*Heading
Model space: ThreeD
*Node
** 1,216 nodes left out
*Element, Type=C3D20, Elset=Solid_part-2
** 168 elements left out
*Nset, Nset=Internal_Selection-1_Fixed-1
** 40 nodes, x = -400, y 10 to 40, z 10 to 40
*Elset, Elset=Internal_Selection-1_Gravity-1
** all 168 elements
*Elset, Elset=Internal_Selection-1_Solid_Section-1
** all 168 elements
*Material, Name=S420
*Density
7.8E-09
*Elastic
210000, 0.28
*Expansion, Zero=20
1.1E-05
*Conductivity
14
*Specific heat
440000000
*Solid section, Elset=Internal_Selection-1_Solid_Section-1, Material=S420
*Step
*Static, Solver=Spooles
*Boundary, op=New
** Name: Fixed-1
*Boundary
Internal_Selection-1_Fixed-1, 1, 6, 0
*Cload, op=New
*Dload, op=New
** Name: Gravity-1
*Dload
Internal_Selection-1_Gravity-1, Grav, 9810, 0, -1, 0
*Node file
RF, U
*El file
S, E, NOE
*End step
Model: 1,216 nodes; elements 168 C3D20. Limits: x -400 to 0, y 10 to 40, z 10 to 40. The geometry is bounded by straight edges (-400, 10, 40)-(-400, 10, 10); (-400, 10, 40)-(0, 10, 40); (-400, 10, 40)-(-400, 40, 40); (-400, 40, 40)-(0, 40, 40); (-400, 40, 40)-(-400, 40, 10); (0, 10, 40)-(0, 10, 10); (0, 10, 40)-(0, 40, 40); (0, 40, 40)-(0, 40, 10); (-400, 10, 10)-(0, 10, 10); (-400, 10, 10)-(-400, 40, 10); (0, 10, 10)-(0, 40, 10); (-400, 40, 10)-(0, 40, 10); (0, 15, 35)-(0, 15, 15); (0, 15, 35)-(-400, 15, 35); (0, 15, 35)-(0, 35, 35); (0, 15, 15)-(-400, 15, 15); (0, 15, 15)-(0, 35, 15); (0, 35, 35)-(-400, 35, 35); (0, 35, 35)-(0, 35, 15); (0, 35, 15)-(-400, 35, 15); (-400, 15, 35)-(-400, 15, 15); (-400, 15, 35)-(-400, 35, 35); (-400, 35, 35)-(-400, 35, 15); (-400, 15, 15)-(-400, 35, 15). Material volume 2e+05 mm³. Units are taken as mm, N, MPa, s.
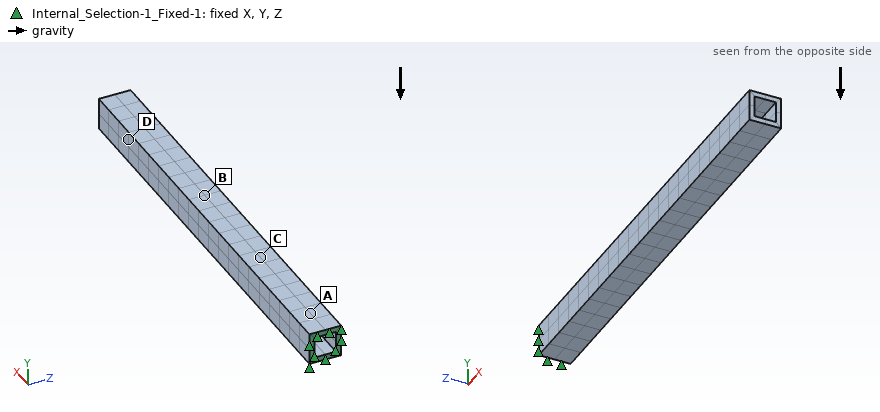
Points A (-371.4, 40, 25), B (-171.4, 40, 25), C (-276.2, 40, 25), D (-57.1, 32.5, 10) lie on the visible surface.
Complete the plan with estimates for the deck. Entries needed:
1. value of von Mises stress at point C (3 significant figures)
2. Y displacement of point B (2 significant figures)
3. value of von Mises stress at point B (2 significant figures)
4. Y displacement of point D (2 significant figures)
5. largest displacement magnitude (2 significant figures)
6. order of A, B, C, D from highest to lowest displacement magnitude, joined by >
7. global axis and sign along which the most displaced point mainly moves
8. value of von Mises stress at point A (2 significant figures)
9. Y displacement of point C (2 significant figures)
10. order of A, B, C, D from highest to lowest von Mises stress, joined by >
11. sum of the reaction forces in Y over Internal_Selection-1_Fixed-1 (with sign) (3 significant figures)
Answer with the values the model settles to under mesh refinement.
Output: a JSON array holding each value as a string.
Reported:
["0.405 MPa", "-0.0048 mm", "0.16 MPa", "-0.0088 mm", "0.011 mm", "D > B > C > A", "-Y", "0.73 MPa", "-0.0017 mm", "A > C > B > D", "15.3 N"]
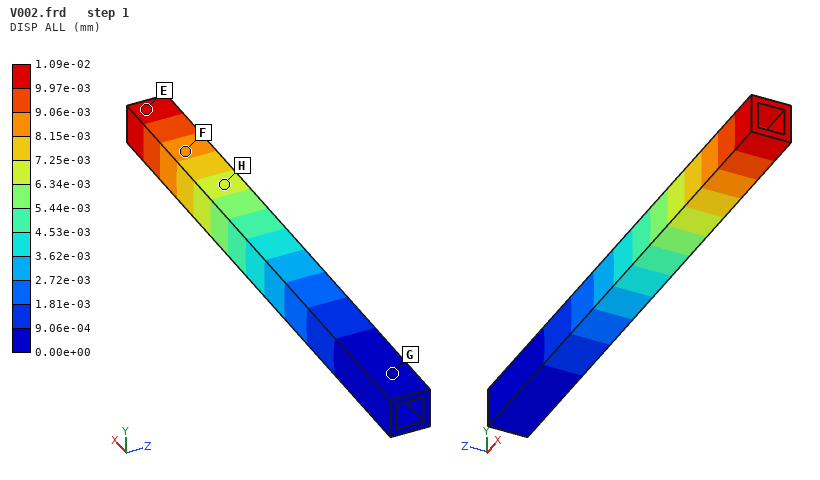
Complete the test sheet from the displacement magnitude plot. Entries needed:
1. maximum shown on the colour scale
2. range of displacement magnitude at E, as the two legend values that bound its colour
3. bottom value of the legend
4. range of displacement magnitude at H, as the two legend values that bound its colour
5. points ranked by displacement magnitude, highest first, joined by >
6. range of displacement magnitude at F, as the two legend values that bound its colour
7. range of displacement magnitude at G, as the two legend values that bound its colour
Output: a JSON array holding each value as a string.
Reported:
["1.09e-02 mm", "9.97e-03 to 1.09e-02 mm", "0.00e+00 mm", "6.34e-03 to 7.25e-03 mm", "E > F > H > G", "8.15e-03 to 9.06e-03 mm", "0.00e+00 to 9.06e-04 mm"]
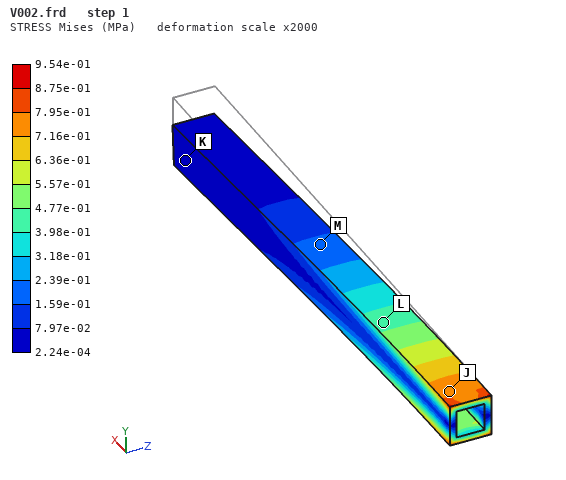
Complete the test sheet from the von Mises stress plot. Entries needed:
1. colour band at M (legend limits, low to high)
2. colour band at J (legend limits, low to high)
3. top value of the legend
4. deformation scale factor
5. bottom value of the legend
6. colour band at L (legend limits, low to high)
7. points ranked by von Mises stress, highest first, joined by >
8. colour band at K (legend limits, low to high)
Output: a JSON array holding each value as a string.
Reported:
["1.59e-01 to 2.39e-01 MPa", "7.16e-01 to 7.95e-01 MPa", "9.54e-01 MPa", "2000", "2.24e-04 MPa", "3.98e-01 to 4.77e-01 MPa", "J > L > M > K", "2.24e-04 to 7.97e-02 MPa"]
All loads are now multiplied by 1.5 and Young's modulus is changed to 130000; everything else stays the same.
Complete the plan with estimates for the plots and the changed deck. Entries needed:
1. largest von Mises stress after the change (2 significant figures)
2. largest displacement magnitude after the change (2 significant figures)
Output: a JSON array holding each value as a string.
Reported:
["1.4 MPa", "0.026 mm"]
